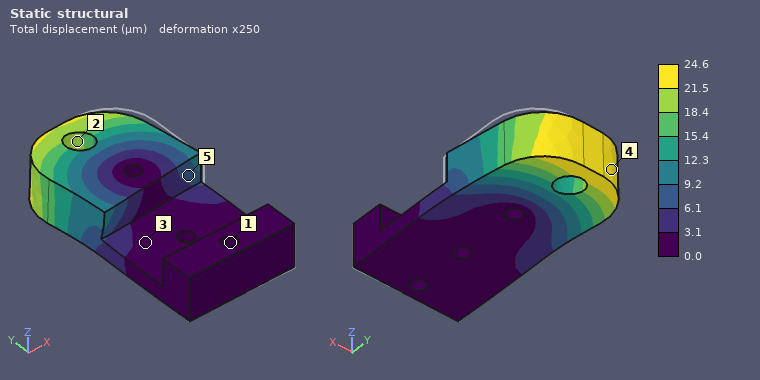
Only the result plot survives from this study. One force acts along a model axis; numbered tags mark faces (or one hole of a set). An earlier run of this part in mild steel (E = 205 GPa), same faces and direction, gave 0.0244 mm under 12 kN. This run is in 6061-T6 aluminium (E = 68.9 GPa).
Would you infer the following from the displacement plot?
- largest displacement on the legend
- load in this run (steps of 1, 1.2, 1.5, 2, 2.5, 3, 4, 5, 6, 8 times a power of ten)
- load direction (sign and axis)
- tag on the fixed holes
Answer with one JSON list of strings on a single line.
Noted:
["24.6 µm", "4 kN", "-X", "1"]
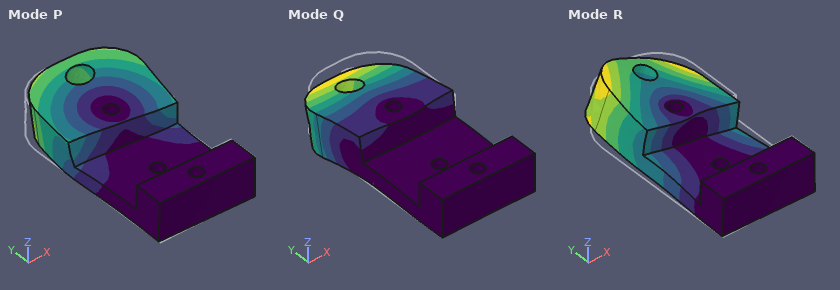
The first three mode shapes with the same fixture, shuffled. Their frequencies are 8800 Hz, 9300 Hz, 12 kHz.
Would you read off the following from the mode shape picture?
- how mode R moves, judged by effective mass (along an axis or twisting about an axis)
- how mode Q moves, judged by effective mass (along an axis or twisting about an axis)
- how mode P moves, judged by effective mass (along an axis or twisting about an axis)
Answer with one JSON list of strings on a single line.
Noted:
["twisting about Y", "along Z", "along X"]
